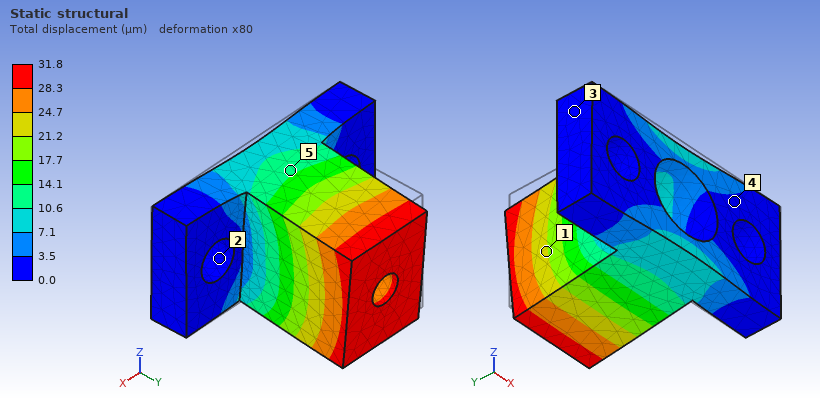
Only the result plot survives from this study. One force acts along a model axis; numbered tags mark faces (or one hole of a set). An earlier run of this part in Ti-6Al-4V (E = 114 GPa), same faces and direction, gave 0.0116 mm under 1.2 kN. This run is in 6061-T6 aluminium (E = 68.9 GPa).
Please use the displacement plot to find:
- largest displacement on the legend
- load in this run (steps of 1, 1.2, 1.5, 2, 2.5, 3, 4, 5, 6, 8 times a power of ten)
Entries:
31.8 µm
2 kN
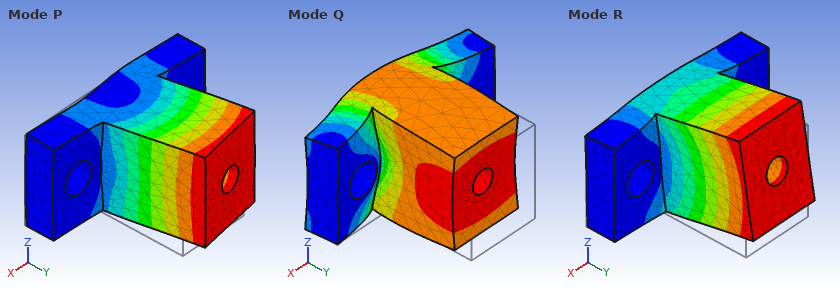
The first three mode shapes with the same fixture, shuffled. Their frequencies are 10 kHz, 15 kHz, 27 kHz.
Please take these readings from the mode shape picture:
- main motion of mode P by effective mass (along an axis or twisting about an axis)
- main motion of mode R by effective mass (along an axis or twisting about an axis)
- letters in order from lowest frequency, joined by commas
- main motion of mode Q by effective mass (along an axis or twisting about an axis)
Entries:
along X
along Z
R, P, Q
along Y
